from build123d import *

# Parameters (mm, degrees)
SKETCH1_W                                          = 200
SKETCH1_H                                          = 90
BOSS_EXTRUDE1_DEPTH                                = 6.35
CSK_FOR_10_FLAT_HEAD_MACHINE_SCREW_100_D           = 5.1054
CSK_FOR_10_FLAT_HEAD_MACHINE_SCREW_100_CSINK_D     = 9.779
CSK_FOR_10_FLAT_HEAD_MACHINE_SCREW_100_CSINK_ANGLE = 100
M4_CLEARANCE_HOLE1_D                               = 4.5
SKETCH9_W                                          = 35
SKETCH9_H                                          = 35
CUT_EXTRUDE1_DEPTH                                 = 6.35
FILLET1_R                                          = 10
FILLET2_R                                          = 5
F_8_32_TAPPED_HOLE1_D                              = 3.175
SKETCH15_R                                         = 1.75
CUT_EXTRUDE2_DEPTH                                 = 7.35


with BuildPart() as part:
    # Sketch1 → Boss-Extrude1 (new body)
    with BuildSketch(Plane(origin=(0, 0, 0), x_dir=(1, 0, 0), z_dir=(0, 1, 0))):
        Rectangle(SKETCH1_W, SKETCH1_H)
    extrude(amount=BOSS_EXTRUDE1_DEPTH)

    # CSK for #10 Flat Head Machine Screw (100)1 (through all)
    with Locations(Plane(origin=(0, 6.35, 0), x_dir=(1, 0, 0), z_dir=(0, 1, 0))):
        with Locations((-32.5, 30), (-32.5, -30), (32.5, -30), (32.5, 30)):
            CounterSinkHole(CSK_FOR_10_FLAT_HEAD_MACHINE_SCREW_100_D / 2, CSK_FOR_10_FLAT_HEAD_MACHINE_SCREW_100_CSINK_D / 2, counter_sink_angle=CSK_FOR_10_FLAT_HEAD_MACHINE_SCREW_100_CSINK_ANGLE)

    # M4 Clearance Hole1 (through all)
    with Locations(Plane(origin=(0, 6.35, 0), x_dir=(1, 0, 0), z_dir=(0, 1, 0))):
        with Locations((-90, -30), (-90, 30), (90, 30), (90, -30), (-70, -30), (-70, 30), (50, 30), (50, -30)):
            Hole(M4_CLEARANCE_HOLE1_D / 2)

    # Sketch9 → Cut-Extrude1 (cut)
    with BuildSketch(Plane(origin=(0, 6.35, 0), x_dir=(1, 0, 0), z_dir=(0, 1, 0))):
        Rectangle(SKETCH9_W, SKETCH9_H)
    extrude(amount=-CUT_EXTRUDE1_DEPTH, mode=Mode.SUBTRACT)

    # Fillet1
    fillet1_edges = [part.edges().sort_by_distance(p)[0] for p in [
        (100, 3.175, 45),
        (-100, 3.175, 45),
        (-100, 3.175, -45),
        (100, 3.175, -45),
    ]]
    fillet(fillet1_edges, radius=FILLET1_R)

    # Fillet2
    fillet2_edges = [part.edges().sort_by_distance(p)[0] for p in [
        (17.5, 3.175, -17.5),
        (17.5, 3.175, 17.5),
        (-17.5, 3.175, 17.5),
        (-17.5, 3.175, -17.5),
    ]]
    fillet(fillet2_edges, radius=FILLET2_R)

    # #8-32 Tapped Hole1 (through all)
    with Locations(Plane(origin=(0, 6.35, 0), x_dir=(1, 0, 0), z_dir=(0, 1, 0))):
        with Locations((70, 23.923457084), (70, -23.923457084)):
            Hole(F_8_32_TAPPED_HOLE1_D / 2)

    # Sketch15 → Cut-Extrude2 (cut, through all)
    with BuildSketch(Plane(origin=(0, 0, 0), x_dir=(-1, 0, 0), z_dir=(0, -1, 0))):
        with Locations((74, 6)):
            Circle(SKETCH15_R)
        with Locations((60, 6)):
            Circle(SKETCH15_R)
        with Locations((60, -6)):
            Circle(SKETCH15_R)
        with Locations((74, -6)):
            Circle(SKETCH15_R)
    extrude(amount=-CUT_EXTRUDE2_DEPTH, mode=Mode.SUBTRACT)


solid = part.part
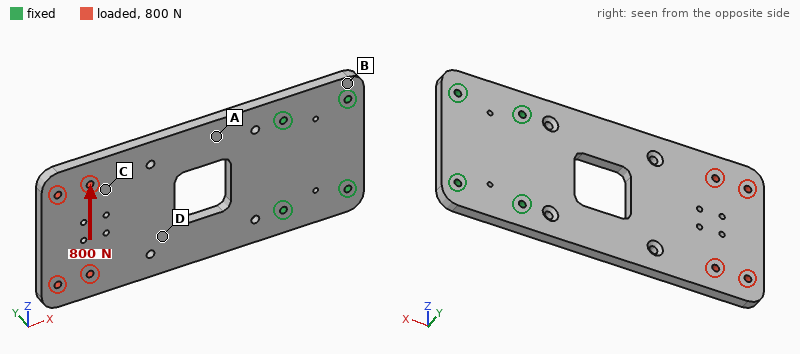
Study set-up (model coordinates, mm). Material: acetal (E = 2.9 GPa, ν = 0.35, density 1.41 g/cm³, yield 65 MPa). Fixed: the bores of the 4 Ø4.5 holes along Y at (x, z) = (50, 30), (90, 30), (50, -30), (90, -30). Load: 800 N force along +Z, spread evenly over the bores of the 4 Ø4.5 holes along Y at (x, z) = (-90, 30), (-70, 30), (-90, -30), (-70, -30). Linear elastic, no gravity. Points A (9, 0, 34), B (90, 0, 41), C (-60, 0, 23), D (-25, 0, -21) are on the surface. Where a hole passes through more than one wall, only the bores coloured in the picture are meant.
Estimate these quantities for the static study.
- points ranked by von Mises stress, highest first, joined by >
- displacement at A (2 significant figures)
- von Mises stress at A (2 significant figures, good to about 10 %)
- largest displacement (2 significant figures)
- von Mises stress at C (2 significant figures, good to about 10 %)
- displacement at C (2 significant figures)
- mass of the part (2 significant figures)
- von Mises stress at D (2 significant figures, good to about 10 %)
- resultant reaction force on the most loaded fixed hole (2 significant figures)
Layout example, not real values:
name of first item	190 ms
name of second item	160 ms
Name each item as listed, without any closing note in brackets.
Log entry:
points ranked by von Mises stress, highest first, joined by >	A > D > C > B
displacement at A	0.32 mm
von Mises stress at A	9.0 MPa
largest displacement	1.3 mm
von Mises stress at C	3.2 MPa
displacement at C	0.97 mm
mass of the part	150 g
von Mises stress at D	6.3 MPa
resultant reaction force on the most loaded fixed hole	1.4 kN
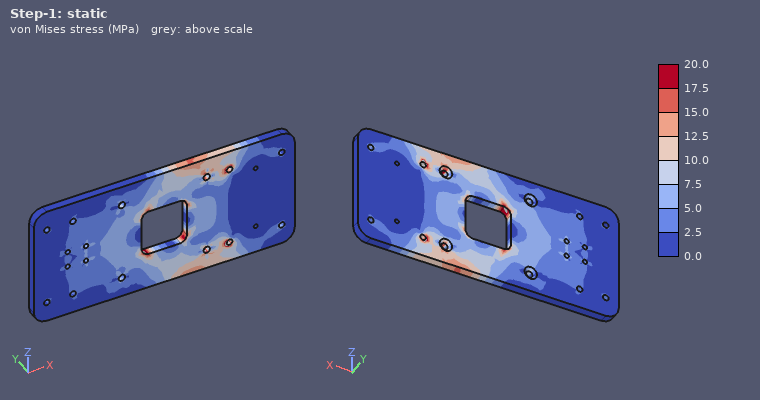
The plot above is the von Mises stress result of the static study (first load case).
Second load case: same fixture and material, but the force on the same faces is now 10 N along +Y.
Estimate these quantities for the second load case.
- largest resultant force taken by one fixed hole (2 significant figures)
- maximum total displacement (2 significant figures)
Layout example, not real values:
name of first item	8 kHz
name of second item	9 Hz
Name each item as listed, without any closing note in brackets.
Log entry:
largest resultant force taken by one fixed hole	12 N
maximum total displacement	2.2 mm
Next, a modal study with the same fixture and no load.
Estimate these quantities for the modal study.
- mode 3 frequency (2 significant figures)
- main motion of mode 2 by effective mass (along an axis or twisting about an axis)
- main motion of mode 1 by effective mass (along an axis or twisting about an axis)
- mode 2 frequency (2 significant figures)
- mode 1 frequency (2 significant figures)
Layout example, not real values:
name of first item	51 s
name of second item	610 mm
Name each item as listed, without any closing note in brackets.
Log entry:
mode 3 frequency	390 Hz
main motion of mode 2 by effective mass	twisting about X
main motion of mode 1 by effective mass	along Y
mode 2 frequency	210 Hz
mode 1 frequency	57 Hz
